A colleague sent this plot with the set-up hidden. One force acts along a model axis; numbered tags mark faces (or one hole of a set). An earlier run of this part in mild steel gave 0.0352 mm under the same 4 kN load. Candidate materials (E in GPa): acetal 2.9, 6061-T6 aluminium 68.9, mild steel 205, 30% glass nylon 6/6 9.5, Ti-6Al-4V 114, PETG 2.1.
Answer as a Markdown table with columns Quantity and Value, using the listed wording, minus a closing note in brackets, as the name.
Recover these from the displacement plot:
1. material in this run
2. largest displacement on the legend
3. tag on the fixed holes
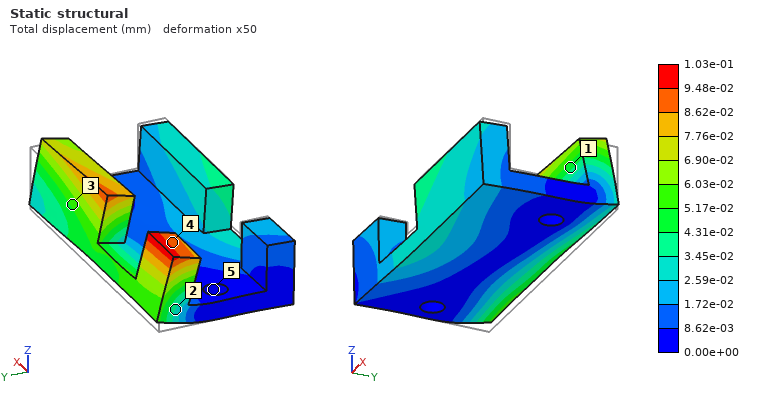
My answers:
| Quantity | Value |
|---|---|
| material in this run | 6061-T6 aluminium |
| largest displacement on the legend | 1.03e-01 mm |
| tag on the fixed holes | 5 |
